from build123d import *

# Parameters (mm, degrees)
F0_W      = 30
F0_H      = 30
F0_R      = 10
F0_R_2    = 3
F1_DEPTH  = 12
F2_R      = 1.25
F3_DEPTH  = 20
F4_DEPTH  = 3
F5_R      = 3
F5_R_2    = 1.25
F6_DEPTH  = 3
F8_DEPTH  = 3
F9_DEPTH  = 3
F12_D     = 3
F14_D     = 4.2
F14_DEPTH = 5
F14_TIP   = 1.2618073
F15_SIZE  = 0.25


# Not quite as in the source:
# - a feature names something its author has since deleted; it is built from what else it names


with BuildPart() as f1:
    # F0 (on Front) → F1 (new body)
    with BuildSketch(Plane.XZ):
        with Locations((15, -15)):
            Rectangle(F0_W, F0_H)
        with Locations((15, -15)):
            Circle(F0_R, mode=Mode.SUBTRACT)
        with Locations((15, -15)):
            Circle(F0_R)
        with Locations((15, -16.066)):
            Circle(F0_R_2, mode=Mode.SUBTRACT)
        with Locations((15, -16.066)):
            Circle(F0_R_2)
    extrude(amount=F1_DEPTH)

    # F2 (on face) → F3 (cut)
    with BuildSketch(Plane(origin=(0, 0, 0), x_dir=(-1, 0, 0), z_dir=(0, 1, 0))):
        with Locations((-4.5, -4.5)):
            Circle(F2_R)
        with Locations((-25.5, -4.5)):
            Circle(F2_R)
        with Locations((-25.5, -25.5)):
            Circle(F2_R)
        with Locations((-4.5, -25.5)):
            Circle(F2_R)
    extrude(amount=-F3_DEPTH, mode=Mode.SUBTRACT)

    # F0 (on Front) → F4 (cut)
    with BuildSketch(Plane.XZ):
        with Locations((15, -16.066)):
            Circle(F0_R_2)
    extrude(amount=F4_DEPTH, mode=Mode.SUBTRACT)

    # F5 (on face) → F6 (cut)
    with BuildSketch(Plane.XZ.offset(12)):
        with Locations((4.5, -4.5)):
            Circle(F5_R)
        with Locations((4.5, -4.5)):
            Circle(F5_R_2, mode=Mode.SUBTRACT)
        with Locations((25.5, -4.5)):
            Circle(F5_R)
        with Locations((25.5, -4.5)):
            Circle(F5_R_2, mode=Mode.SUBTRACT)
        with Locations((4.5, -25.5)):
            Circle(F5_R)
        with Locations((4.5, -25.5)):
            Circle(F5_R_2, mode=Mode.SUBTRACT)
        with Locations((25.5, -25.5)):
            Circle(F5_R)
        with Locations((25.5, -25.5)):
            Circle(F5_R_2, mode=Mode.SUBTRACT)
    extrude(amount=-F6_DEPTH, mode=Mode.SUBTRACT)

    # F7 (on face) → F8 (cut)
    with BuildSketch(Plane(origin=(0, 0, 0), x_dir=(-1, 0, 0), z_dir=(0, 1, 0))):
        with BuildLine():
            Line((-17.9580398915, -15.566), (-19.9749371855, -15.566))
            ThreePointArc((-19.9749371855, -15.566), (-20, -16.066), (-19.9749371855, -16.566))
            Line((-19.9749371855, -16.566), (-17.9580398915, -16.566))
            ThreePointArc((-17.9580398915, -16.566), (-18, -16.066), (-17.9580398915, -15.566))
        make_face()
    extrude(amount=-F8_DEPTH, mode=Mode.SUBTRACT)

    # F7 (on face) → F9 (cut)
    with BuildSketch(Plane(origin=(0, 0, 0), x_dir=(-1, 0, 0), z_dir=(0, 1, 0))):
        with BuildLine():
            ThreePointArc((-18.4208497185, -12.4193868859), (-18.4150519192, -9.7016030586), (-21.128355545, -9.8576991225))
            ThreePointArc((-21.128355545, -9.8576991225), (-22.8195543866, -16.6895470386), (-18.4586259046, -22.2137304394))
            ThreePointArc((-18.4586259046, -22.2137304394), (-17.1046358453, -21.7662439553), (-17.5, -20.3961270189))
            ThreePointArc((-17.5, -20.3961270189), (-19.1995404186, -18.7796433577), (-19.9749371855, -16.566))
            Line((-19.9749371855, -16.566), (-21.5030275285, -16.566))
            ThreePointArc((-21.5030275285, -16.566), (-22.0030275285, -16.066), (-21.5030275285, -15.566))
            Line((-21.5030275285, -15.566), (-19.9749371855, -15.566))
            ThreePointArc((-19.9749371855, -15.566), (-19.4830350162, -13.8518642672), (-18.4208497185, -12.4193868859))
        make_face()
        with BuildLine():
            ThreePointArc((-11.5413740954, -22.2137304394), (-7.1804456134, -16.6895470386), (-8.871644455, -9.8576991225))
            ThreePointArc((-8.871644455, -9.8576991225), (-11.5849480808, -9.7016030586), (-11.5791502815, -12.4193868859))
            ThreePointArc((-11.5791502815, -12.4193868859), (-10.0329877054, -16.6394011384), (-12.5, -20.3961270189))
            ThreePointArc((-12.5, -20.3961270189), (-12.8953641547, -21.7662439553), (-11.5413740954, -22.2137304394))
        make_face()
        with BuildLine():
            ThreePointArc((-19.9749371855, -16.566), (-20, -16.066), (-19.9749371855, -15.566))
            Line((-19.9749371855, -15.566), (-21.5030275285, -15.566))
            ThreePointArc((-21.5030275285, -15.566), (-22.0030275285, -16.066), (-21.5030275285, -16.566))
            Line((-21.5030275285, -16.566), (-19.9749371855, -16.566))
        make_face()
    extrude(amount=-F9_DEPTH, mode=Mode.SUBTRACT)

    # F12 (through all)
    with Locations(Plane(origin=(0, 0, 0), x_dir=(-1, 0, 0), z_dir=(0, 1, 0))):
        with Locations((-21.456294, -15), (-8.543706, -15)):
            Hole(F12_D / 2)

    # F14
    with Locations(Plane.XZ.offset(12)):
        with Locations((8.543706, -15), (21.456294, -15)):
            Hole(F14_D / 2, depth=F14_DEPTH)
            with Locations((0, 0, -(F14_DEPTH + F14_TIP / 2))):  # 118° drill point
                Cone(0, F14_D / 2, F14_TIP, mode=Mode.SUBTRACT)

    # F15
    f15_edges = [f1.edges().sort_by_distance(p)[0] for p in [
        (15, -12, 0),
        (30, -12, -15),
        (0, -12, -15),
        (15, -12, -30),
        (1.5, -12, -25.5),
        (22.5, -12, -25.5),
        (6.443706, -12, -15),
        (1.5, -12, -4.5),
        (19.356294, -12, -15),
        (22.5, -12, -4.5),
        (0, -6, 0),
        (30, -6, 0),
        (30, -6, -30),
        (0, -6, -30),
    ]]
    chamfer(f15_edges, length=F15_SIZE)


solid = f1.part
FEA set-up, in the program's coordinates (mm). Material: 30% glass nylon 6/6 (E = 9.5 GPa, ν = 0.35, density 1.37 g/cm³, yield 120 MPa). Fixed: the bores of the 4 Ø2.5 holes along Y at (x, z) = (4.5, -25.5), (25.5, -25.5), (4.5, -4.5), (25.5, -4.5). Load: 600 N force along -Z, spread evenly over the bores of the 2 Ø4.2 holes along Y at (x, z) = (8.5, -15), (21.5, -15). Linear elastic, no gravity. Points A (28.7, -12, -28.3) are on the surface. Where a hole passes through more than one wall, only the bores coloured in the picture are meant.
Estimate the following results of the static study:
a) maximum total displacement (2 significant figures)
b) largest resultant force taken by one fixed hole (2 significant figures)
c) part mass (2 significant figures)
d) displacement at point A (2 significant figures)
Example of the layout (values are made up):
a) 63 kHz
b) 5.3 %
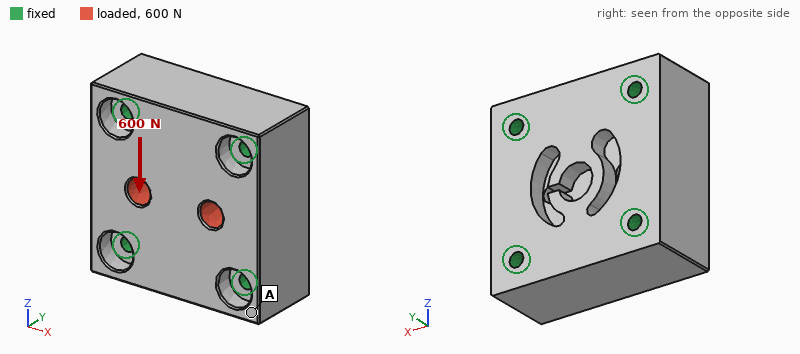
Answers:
a) 4.4 µm
b) 170 N
c) 13 g
d) 0.93 µm
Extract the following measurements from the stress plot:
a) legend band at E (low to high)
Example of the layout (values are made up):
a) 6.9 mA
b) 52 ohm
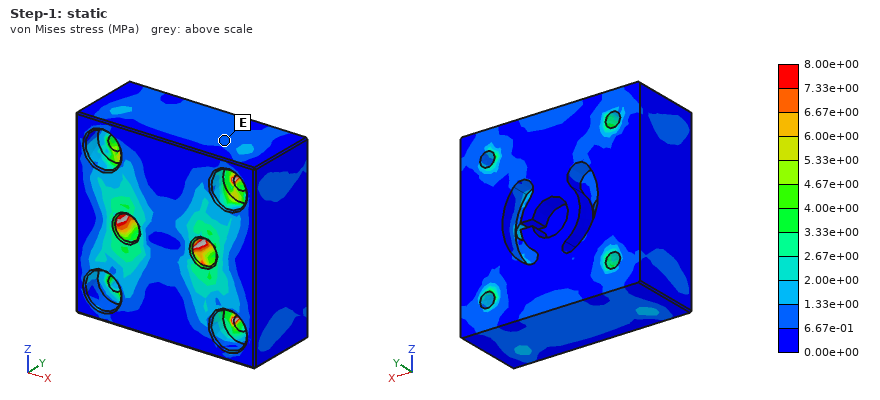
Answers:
a) 6.67e-01 to 1.33e+00 MPa
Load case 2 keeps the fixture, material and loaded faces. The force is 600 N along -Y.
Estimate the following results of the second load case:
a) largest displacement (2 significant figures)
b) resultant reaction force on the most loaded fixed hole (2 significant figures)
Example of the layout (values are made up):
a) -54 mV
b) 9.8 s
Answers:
a) 9.1 µm
b) 160 N
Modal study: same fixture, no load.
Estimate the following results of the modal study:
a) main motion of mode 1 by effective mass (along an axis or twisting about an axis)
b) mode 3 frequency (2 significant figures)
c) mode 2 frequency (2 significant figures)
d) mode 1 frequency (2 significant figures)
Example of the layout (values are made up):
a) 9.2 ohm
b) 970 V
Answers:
a) along Y
b) 29 kHz
c) 28 kHz
d) 22 kHz
